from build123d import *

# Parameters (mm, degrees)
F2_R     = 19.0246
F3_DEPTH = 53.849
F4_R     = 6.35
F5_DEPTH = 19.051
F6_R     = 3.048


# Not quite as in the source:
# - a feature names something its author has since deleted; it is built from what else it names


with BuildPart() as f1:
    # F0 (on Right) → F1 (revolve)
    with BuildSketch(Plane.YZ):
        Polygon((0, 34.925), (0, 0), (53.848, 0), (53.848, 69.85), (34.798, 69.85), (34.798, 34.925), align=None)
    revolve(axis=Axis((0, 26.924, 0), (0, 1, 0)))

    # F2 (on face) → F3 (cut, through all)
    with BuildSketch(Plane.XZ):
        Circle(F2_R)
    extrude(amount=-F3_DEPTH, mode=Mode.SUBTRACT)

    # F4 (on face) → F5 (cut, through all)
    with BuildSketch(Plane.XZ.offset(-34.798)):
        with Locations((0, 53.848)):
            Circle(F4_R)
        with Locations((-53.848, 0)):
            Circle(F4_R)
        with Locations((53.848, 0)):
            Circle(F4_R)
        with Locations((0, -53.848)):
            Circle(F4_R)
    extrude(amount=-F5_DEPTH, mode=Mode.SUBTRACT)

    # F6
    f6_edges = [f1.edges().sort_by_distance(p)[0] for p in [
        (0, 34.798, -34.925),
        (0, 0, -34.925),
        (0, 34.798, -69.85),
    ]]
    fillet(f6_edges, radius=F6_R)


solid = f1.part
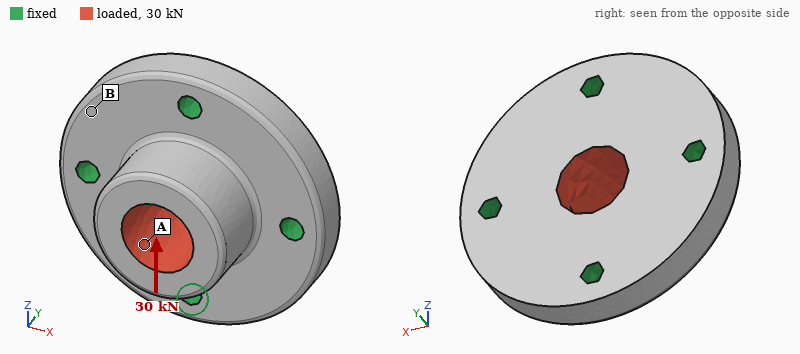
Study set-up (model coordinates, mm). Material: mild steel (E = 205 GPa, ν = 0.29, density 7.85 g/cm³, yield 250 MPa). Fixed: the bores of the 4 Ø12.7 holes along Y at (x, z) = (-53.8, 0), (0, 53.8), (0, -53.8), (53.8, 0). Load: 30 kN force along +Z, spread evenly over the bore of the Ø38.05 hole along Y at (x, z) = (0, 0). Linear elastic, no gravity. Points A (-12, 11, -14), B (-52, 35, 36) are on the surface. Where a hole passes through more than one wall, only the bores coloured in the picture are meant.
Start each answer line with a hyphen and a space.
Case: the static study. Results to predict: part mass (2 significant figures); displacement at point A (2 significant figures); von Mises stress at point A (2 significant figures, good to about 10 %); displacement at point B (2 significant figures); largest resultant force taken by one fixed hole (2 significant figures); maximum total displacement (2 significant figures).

- 2.8 kg
- 6.6 µm
- 12 MPa
- 1.5 µm
- 11 kN
- 8.5 µm
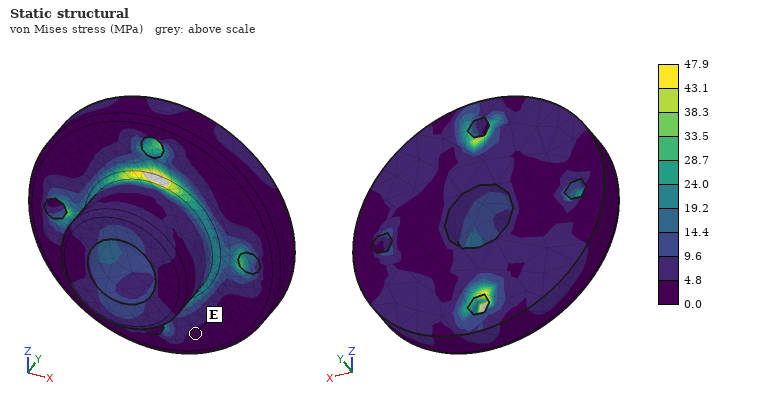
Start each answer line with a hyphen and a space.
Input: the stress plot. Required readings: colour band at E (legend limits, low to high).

- 0.0 to 4.8 MPa
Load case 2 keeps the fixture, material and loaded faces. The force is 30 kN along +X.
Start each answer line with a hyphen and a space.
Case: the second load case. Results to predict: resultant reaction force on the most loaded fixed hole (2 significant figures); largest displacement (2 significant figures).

- 11 kN
- 8.5 µm
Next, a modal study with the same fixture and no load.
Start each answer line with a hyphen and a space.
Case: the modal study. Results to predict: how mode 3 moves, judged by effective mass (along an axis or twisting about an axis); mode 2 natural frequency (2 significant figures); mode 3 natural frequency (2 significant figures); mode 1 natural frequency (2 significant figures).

- along Y
- 9300 Hz
- 9800 Hz
- 9300 Hz
